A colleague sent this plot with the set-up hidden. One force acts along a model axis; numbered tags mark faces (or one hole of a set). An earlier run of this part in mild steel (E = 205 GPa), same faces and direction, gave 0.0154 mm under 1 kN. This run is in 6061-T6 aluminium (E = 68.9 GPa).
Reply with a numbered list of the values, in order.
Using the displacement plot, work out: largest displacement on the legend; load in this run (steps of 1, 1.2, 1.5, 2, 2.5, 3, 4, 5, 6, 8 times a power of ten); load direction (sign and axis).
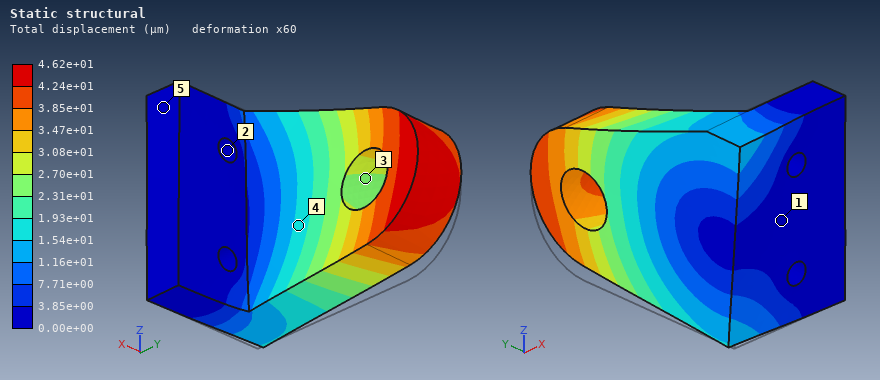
1. 4.62e+01 µm
2. 1 kN
3. +Z
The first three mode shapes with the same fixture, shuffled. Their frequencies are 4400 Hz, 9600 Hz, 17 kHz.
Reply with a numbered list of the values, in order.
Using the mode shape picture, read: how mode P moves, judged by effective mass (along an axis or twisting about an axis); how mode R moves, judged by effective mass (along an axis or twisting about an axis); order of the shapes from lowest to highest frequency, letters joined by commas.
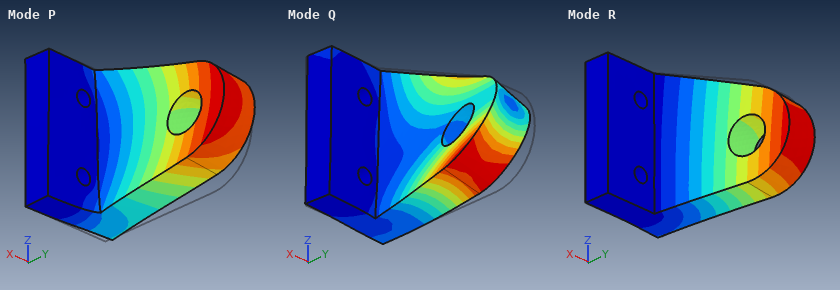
1. along Z
2. along X
3. R, P, Q
